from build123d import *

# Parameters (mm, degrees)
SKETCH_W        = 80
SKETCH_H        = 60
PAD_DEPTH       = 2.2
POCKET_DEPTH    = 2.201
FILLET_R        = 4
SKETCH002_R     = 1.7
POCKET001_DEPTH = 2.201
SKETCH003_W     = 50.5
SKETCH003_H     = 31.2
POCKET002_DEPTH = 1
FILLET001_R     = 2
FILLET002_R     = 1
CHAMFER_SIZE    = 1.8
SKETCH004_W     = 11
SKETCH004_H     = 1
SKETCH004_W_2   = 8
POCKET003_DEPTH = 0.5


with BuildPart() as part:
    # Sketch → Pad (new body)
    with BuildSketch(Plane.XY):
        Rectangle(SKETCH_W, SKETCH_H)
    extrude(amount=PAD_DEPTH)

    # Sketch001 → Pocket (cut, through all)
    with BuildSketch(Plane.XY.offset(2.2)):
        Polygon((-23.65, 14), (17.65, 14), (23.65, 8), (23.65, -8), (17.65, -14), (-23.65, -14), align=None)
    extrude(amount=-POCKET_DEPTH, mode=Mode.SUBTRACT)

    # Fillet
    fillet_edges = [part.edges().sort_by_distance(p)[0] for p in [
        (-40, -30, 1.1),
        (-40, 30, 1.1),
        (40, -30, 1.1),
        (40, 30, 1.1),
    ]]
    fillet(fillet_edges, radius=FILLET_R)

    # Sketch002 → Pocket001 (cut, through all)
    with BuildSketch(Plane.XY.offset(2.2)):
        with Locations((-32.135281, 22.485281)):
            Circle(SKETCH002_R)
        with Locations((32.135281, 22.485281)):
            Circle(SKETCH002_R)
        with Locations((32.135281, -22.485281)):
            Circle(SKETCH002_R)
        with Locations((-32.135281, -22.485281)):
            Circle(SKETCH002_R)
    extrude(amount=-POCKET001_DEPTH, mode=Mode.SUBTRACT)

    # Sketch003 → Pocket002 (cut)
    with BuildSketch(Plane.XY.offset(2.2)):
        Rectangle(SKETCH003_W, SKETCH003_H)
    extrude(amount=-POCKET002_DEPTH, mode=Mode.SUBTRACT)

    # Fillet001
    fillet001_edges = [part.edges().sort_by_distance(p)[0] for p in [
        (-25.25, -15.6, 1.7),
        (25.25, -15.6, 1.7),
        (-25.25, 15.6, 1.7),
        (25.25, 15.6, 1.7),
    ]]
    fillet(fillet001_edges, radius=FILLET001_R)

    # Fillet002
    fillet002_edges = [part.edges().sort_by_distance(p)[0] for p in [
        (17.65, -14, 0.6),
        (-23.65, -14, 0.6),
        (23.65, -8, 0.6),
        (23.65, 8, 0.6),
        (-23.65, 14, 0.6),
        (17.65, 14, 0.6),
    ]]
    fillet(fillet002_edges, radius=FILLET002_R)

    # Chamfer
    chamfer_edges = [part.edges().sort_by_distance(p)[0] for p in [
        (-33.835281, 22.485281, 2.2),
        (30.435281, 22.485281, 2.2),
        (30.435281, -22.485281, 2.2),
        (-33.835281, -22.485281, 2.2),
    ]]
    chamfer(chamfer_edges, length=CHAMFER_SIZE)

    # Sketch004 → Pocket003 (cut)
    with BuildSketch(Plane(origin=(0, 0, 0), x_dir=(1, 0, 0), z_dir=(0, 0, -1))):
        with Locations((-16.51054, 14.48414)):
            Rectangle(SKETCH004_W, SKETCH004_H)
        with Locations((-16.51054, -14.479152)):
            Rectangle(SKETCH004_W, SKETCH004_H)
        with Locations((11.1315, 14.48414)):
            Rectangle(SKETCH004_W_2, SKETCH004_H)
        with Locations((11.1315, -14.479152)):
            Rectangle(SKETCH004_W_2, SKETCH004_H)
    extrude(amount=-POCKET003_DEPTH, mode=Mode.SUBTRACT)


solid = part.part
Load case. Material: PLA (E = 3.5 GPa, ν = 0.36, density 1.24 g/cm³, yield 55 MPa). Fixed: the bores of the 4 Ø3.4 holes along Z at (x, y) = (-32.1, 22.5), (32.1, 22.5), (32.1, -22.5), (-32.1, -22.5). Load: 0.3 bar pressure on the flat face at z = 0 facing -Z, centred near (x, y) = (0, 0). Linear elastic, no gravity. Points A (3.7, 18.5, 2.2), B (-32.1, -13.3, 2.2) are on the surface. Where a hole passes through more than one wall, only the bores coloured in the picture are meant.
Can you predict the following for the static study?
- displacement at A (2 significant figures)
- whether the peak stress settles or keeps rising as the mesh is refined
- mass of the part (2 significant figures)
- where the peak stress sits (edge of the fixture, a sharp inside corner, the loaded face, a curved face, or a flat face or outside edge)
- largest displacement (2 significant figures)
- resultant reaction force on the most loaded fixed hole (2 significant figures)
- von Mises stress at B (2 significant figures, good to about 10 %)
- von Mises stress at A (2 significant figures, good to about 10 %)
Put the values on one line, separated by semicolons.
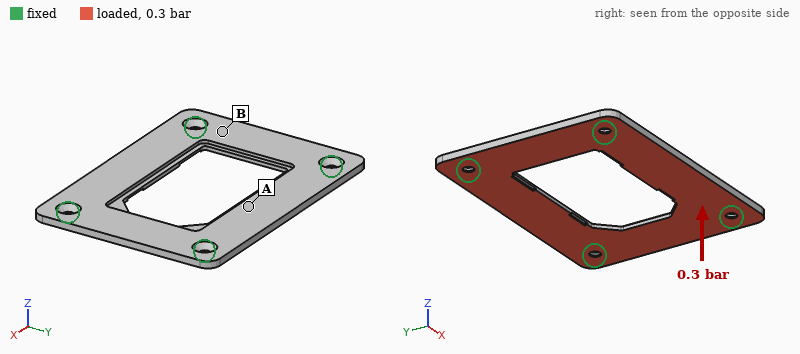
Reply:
0.64 mm; keeps rising; 9.0 g; edge of the fixture; 0.71 mm; 60 N; 4.2 MPa; 9.3 MPa
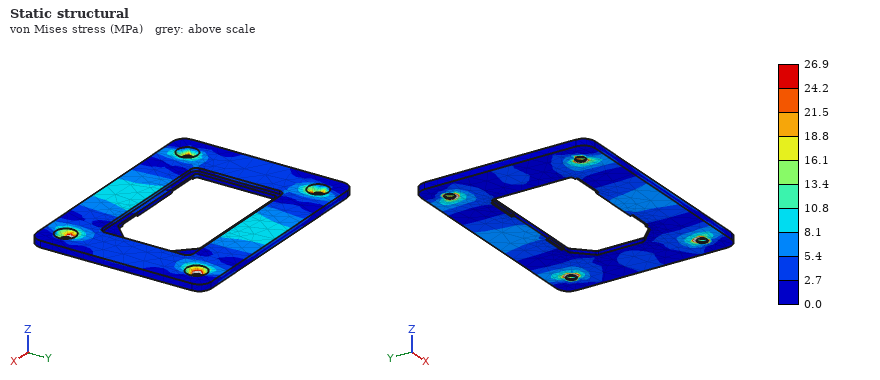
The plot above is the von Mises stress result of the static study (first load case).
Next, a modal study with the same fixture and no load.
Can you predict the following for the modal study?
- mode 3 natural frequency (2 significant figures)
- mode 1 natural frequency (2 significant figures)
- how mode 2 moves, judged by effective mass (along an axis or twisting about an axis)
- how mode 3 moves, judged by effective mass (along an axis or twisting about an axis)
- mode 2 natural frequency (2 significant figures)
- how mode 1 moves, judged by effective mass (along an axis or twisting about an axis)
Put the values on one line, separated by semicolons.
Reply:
1400 Hz; 760 Hz; twisting about X; along Z; 820 Hz; along Z
